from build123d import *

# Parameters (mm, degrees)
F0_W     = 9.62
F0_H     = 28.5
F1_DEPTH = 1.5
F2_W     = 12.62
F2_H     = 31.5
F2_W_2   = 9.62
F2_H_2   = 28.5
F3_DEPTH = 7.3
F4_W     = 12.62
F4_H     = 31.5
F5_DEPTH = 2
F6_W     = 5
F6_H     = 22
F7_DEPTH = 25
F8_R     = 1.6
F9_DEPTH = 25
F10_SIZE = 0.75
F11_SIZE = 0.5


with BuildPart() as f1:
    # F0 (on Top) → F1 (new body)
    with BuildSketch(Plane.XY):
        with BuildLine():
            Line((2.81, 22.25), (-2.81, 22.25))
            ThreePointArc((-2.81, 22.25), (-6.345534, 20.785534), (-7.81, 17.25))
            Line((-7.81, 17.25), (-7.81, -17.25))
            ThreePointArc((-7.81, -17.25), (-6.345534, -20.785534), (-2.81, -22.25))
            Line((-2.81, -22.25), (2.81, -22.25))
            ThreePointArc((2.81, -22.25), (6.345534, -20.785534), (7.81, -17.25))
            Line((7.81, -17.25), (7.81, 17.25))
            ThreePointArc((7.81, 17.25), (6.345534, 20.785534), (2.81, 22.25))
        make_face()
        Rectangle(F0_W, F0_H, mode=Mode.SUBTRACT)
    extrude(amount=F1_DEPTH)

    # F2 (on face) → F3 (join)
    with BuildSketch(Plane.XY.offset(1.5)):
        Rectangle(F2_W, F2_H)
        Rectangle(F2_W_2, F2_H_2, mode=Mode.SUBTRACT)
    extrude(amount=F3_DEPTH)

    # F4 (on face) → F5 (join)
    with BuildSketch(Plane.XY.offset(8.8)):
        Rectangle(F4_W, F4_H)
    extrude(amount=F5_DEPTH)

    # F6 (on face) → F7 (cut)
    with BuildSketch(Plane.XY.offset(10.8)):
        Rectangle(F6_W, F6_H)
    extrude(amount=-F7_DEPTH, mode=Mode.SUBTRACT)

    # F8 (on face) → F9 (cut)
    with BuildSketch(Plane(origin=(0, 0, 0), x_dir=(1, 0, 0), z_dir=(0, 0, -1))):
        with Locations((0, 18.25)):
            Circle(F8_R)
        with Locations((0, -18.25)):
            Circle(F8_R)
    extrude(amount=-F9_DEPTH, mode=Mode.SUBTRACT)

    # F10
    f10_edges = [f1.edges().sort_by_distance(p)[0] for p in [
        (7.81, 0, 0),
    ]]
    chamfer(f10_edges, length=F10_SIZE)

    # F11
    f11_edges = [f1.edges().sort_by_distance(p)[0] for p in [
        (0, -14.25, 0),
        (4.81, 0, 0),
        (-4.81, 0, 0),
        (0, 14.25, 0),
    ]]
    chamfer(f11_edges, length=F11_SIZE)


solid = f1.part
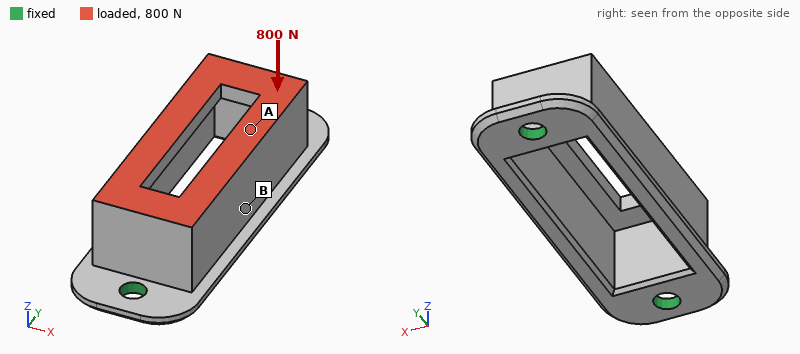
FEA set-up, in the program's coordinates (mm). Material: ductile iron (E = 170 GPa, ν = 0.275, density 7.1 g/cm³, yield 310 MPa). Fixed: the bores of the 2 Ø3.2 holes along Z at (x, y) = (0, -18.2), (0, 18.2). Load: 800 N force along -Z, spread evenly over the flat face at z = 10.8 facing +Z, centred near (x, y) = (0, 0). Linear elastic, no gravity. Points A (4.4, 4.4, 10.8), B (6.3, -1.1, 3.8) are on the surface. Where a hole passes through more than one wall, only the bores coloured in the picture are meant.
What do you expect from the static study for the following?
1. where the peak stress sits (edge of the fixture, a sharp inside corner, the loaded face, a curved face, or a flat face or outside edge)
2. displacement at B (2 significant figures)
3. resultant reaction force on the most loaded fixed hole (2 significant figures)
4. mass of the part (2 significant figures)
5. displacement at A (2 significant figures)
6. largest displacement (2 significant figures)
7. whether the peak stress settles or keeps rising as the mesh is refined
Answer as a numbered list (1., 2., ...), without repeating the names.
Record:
1. edge of the fixture
2. 6.7 µm
3. 440 N
4. 14 g
5. 7.5 µm
6. 9.3 µm
7. keeps rising
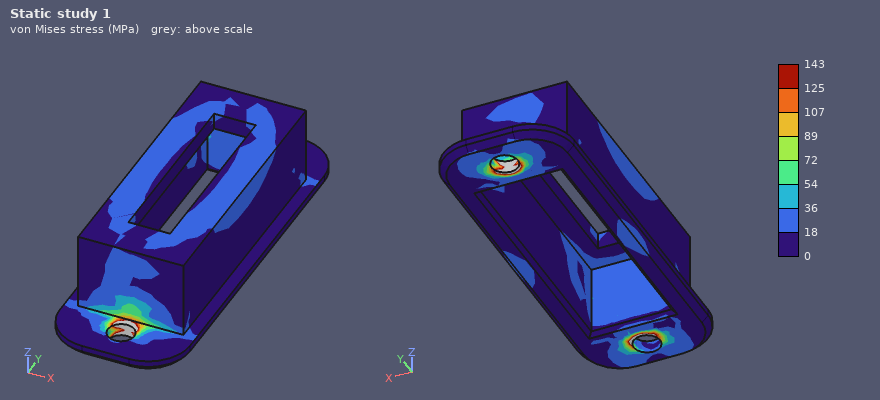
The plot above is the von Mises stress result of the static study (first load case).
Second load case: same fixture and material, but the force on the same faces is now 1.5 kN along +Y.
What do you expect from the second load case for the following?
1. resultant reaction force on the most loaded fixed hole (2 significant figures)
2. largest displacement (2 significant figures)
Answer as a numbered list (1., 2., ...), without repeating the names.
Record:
1. 880 N
2. 11 µm
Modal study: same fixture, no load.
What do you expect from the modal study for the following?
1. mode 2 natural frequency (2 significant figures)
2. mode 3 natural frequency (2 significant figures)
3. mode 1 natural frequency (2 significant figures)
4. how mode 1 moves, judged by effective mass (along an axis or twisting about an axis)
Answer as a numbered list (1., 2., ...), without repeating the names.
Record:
1. 13 kHz
2. 13 kHz
3. 6100 Hz
4. along X
